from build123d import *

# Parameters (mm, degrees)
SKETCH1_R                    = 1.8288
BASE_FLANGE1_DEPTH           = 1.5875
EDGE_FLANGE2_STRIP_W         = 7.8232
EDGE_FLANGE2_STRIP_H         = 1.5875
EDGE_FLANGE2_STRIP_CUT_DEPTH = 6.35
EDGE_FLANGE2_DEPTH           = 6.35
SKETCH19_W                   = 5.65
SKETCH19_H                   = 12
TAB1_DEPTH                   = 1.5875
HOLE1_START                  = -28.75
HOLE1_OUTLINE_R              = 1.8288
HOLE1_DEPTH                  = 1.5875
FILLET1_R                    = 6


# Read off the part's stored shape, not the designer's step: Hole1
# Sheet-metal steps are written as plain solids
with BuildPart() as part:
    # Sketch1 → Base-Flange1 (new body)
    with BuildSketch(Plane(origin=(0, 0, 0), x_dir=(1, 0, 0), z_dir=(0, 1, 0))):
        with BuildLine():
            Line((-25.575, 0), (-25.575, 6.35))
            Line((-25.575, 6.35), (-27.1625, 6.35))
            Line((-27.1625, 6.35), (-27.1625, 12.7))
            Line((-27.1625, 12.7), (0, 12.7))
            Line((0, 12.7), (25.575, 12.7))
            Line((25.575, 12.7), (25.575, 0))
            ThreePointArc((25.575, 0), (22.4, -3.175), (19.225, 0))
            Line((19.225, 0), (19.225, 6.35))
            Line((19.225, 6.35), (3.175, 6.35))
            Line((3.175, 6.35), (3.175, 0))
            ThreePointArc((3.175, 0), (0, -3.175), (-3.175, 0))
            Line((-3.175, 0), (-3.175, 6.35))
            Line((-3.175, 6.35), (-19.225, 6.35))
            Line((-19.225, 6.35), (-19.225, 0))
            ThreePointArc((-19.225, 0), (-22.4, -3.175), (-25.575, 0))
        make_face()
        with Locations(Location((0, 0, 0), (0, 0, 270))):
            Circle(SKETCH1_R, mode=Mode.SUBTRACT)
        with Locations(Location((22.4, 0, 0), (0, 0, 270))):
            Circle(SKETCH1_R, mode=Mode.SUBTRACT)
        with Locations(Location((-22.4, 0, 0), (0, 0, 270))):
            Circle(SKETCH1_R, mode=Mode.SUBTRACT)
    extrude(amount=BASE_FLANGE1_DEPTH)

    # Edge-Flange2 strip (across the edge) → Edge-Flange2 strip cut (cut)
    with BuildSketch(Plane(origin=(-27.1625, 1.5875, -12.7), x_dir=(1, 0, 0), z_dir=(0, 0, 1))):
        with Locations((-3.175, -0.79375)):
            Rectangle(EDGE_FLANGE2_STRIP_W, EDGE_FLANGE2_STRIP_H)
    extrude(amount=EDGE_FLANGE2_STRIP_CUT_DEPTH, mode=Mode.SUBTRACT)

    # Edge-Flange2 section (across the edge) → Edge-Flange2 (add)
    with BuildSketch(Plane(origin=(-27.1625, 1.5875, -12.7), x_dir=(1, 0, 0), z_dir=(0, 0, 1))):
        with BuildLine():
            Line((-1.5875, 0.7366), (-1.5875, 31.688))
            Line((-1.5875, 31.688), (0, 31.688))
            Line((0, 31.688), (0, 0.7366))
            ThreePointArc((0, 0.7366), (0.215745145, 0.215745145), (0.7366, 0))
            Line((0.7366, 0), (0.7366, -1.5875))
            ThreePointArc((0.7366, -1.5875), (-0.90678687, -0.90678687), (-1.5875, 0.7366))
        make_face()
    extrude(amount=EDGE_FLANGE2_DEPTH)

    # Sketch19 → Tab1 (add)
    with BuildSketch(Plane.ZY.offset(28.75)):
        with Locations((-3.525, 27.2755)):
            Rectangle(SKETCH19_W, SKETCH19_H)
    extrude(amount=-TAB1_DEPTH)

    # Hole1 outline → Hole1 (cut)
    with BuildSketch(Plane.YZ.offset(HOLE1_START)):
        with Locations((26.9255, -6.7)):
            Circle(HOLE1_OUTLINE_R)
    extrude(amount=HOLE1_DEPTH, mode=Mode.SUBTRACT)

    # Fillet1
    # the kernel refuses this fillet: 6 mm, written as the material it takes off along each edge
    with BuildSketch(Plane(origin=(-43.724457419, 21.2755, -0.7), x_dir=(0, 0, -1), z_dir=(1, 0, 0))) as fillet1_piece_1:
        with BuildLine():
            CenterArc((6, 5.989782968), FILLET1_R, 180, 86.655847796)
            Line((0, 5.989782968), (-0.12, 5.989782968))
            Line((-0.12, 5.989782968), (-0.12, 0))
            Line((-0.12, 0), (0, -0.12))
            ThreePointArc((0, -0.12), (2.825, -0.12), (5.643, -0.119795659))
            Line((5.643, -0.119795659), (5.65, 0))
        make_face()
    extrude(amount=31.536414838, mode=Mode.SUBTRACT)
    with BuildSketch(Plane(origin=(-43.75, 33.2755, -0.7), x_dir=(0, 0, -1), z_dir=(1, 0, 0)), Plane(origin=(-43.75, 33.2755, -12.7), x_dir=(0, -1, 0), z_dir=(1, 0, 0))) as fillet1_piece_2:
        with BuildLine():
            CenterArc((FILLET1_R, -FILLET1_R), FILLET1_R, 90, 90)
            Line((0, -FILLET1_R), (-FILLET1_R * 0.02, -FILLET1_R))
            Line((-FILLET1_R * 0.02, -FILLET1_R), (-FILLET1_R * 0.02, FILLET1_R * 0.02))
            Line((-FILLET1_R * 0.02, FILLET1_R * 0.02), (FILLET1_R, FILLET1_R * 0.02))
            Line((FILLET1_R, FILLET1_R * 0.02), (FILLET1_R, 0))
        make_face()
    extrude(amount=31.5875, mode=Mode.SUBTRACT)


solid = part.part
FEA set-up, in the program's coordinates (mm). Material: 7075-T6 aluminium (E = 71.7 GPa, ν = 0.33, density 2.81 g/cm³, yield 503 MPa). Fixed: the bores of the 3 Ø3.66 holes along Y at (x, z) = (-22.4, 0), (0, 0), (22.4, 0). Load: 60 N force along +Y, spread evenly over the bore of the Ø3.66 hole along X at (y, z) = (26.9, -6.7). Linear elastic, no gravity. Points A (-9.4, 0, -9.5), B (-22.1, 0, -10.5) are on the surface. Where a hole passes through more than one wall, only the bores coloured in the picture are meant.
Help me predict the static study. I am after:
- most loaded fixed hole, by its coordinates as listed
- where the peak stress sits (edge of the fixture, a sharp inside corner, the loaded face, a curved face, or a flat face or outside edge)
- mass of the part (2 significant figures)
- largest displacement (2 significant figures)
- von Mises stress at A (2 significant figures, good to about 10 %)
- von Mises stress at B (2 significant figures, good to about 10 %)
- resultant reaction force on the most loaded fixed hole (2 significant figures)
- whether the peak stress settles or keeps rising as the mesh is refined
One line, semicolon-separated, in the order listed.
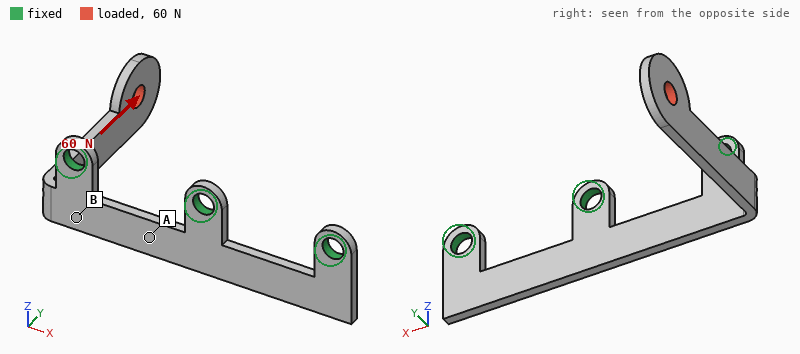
(-22.4, 0); a sharp inside corner; 3.2 g; 0.34 mm; 16 MPa; 42 MPa; 65 N; keeps rising
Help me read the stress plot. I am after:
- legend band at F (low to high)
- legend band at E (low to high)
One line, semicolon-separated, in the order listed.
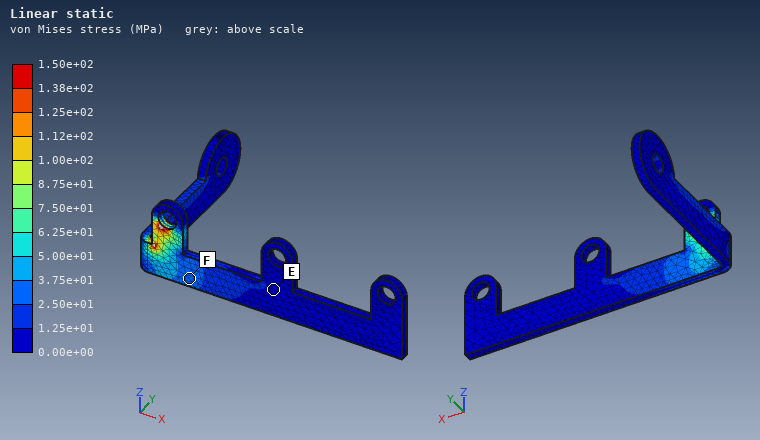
2.50e+01 to 3.75e+01 MPa; 0.00e+00 to 1.25e+01 MPa
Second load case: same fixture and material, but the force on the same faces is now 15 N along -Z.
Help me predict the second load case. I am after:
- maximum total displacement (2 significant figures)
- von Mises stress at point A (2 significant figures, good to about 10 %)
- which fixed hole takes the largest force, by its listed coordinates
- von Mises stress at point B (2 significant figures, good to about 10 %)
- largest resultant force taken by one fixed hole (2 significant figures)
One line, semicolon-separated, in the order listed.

0.70 mm; 33 MPa; (-22.4, 0); 73 MPa; 18 N
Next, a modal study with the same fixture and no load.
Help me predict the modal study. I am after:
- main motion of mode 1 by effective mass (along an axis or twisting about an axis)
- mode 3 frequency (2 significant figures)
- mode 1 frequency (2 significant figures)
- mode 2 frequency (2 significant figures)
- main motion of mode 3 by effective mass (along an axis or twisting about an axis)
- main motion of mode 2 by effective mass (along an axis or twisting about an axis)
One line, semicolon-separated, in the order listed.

along X; 4700 Hz; 780 Hz; 1000 Hz; along Y; along Z
